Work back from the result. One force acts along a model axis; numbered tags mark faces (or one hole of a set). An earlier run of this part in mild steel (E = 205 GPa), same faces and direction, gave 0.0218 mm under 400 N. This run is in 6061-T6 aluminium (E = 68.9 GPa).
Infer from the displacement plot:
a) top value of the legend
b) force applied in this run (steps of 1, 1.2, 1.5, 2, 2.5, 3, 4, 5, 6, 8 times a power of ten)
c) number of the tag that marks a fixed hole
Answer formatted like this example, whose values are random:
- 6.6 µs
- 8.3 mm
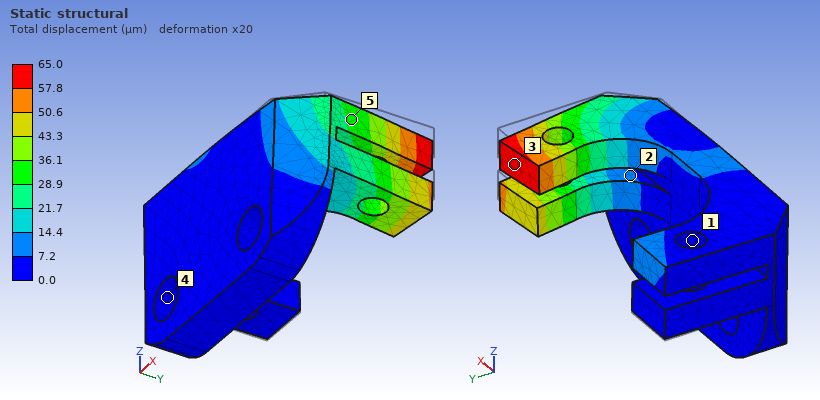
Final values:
- 65.0 µm
- 400 N
- 4
